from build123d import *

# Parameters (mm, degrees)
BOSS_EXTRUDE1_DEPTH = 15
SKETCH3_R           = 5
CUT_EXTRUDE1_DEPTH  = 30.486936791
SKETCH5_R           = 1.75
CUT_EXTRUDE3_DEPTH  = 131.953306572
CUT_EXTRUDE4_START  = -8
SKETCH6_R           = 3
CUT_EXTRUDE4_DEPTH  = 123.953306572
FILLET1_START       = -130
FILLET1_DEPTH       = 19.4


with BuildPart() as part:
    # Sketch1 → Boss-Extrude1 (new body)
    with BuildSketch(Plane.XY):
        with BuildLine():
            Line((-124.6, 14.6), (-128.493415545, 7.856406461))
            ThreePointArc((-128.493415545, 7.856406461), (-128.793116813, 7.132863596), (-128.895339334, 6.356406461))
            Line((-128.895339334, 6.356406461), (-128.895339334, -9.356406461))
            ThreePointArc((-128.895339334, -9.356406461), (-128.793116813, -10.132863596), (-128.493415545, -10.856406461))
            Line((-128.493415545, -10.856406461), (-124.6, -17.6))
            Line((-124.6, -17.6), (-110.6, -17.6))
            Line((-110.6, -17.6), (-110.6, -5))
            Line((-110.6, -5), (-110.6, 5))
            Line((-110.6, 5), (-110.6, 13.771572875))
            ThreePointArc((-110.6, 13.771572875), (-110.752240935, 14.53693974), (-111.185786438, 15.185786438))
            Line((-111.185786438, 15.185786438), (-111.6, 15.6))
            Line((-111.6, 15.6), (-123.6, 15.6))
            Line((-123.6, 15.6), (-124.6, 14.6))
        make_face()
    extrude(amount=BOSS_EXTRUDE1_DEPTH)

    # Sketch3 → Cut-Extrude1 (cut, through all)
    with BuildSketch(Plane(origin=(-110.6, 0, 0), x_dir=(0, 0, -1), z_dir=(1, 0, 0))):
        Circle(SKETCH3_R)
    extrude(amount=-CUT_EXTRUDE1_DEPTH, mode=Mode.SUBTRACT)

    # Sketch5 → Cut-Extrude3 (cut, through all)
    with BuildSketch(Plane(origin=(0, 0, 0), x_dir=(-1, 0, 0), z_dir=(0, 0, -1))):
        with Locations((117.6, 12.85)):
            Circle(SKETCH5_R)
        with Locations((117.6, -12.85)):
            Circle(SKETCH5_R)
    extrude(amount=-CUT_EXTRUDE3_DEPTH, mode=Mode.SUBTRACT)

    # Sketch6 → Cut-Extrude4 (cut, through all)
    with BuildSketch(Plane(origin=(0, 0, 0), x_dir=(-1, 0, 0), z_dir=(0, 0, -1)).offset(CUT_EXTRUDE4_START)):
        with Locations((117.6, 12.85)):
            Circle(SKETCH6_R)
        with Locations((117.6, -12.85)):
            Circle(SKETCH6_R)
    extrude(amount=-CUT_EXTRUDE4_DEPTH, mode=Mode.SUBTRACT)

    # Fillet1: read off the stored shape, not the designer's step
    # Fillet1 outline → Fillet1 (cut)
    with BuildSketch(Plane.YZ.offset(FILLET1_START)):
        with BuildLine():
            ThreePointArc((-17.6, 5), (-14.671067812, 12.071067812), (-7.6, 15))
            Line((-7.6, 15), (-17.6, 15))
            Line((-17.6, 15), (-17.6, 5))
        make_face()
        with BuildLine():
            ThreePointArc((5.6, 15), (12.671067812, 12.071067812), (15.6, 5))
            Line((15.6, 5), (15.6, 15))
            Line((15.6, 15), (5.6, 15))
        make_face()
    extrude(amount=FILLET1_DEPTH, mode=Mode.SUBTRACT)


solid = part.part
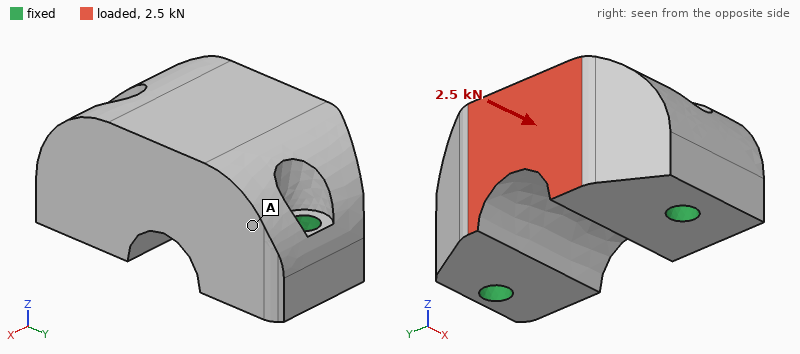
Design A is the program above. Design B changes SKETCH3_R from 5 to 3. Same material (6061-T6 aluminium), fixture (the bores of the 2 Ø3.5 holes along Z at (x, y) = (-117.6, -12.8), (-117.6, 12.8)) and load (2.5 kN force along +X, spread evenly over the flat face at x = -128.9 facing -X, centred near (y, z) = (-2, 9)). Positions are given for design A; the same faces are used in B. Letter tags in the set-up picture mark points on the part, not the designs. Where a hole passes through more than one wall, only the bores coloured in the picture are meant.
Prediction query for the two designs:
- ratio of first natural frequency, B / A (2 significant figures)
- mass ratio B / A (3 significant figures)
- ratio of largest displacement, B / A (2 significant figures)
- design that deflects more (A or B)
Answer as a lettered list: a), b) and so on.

a) 0.99
b) 1.07
c) 0.84
d) A
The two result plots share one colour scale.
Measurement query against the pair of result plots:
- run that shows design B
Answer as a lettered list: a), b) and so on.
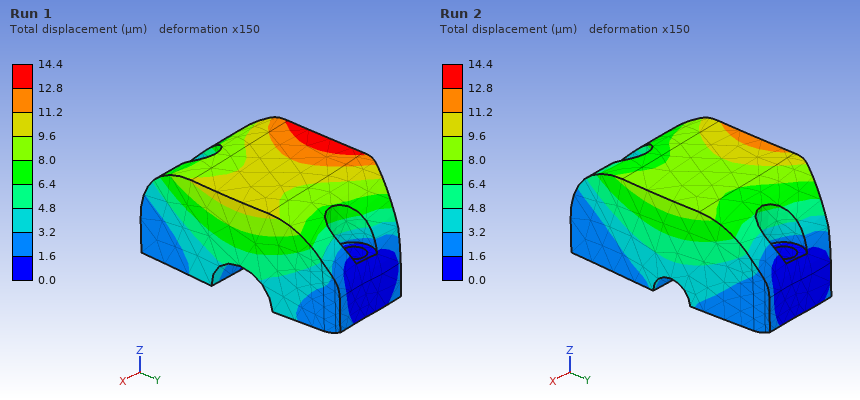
a) Run 2
